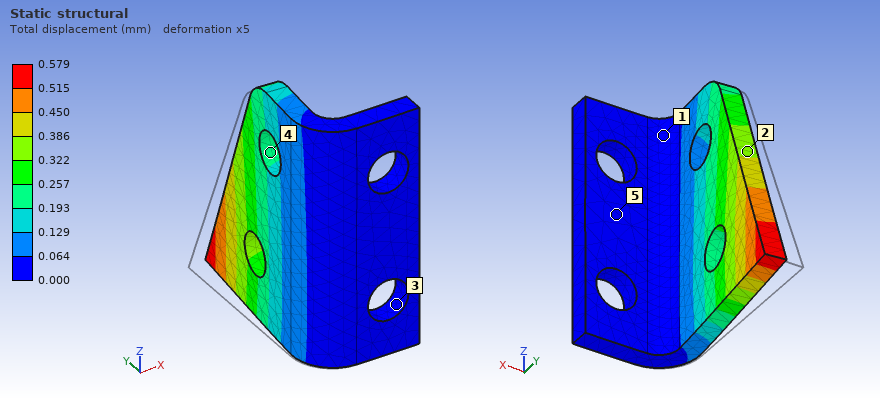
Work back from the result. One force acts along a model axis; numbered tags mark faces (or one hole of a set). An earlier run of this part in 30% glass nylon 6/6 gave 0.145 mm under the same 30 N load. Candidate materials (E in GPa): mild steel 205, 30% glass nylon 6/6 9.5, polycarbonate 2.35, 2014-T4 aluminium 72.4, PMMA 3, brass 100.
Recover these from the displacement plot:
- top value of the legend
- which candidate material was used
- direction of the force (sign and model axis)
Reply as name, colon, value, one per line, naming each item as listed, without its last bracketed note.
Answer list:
top value of the legend: 0.579 mm
which candidate material was used: polycarbonate
direction of the force: +X
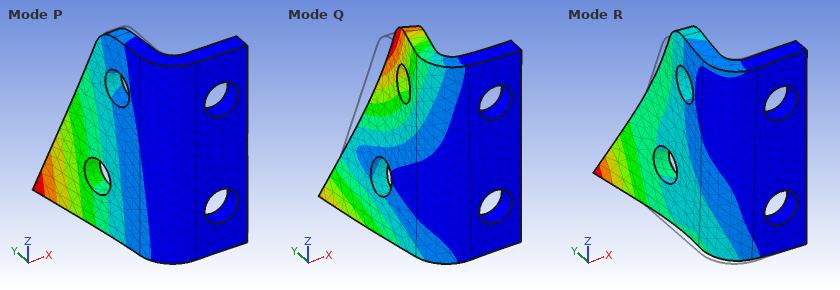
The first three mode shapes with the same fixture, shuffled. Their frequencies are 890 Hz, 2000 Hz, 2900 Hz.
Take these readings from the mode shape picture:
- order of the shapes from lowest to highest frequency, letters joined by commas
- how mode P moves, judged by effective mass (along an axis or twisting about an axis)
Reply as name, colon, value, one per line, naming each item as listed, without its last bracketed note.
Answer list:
order of the shapes from lowest to highest frequency, letters joined by commas: P, Q, R
how mode P moves, judged by effective mass: along X
